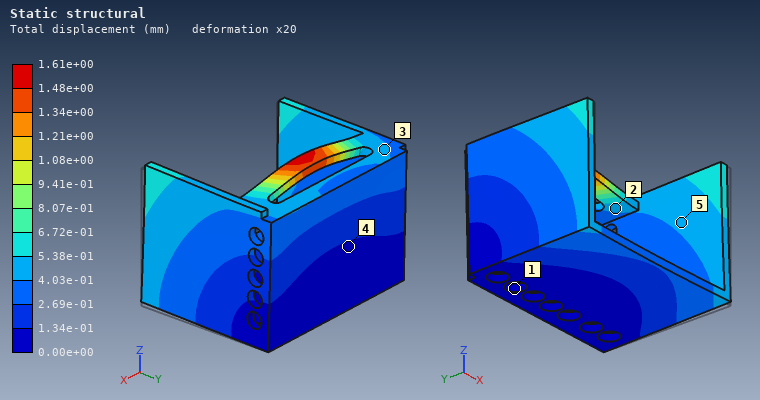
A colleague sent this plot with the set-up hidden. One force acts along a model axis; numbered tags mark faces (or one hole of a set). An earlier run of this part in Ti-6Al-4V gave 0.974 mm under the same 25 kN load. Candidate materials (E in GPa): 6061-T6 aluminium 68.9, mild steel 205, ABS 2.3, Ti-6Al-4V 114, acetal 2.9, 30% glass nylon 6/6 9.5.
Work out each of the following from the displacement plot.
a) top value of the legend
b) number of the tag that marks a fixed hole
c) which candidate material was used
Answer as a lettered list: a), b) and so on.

a) 1.61e+00 mm
b) 1
c) 6061-T6 aluminium
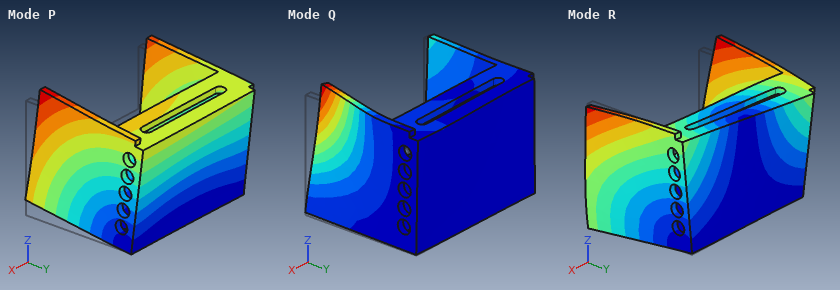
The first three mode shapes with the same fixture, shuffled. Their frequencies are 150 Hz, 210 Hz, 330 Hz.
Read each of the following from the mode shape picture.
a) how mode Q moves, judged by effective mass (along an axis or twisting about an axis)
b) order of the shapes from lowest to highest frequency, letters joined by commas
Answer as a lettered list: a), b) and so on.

a) along X
b) P, R, Q
